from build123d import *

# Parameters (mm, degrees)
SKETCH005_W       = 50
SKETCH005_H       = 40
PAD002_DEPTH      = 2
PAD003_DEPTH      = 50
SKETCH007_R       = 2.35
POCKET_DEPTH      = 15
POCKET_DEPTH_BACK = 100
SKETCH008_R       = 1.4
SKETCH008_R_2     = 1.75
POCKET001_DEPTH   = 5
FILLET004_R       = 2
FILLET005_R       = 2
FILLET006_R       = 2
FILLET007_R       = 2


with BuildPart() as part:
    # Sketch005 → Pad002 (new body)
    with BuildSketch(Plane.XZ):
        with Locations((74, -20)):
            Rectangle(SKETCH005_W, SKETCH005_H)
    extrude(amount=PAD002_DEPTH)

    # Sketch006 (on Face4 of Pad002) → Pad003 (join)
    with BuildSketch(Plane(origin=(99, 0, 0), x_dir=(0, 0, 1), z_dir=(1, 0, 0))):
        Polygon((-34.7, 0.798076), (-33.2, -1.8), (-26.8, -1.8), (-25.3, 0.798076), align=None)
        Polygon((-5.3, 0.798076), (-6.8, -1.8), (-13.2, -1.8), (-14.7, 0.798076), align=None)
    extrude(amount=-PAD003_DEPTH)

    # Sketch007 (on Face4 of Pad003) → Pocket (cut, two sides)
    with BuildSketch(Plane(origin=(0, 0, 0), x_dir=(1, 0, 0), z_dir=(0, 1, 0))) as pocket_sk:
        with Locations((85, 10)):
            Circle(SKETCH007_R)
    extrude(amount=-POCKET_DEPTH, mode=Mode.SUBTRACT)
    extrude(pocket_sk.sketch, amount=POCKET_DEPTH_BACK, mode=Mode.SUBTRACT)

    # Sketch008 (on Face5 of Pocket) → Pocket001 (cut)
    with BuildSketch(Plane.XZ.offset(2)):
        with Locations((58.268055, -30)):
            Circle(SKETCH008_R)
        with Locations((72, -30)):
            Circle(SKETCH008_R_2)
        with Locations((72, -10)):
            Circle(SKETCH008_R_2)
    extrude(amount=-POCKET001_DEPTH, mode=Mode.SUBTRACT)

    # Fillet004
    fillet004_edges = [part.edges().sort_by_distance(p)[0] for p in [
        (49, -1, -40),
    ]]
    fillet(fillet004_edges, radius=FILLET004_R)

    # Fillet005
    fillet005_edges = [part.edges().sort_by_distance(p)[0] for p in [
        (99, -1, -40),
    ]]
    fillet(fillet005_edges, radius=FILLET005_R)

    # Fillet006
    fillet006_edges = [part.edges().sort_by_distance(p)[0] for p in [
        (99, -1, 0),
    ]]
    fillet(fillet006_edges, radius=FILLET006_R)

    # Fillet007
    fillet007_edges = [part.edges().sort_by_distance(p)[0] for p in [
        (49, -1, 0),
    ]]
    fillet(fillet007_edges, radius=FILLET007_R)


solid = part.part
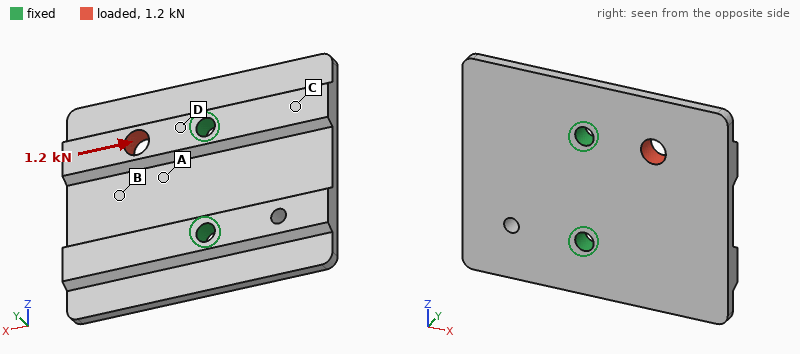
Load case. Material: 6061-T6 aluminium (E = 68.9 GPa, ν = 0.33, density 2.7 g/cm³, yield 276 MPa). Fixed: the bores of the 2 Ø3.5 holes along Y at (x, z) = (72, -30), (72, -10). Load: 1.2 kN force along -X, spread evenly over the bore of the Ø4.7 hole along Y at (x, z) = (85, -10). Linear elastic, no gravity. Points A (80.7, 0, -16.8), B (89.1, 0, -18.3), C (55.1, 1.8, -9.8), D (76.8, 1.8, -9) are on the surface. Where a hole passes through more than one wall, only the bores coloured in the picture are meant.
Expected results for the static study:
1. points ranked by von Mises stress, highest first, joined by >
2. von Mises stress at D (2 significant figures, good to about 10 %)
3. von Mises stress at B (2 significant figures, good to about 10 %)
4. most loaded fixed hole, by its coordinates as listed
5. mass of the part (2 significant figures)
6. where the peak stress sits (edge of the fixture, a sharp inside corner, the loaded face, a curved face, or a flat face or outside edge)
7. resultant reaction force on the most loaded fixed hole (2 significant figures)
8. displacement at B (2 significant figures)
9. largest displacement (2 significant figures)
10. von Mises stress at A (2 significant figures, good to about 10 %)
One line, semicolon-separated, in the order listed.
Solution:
D > A > B > C; 44 MPa; 12 MPa; (72, -10); 14 g; the loaded face; 1.2 kN; 8.4 µm; 27 µm; 17 MPa
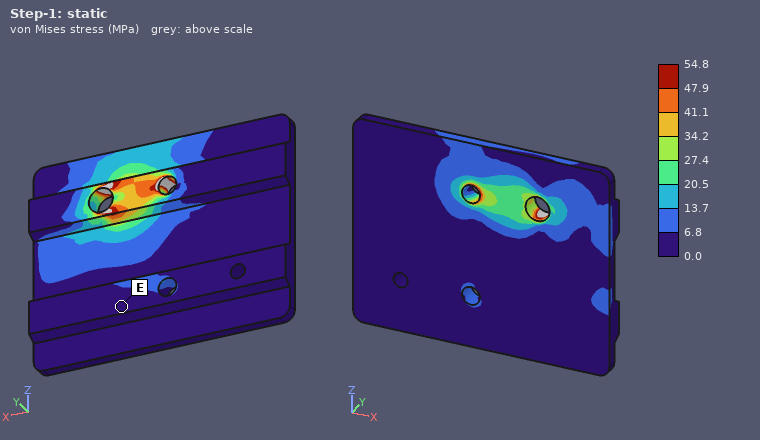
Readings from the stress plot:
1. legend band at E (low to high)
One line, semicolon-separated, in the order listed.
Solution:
0.0 to 6.8 MPa
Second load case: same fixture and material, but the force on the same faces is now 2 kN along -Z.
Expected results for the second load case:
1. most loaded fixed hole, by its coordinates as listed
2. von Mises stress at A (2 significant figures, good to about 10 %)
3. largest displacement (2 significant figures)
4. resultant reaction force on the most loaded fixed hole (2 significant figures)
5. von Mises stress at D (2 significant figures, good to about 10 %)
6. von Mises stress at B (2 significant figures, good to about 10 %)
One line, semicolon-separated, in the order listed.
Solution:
(72, -10); 79 MPa; 53 µm; 1.6 kN; 62 MPa; 55 MPa
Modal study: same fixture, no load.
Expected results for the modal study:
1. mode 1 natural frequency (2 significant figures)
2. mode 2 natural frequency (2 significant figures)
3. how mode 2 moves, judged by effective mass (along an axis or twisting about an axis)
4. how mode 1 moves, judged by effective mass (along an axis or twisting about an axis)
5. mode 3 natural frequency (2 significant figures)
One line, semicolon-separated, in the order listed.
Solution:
3800 Hz; 5400 Hz; along Y; along Y; 5900 Hz
